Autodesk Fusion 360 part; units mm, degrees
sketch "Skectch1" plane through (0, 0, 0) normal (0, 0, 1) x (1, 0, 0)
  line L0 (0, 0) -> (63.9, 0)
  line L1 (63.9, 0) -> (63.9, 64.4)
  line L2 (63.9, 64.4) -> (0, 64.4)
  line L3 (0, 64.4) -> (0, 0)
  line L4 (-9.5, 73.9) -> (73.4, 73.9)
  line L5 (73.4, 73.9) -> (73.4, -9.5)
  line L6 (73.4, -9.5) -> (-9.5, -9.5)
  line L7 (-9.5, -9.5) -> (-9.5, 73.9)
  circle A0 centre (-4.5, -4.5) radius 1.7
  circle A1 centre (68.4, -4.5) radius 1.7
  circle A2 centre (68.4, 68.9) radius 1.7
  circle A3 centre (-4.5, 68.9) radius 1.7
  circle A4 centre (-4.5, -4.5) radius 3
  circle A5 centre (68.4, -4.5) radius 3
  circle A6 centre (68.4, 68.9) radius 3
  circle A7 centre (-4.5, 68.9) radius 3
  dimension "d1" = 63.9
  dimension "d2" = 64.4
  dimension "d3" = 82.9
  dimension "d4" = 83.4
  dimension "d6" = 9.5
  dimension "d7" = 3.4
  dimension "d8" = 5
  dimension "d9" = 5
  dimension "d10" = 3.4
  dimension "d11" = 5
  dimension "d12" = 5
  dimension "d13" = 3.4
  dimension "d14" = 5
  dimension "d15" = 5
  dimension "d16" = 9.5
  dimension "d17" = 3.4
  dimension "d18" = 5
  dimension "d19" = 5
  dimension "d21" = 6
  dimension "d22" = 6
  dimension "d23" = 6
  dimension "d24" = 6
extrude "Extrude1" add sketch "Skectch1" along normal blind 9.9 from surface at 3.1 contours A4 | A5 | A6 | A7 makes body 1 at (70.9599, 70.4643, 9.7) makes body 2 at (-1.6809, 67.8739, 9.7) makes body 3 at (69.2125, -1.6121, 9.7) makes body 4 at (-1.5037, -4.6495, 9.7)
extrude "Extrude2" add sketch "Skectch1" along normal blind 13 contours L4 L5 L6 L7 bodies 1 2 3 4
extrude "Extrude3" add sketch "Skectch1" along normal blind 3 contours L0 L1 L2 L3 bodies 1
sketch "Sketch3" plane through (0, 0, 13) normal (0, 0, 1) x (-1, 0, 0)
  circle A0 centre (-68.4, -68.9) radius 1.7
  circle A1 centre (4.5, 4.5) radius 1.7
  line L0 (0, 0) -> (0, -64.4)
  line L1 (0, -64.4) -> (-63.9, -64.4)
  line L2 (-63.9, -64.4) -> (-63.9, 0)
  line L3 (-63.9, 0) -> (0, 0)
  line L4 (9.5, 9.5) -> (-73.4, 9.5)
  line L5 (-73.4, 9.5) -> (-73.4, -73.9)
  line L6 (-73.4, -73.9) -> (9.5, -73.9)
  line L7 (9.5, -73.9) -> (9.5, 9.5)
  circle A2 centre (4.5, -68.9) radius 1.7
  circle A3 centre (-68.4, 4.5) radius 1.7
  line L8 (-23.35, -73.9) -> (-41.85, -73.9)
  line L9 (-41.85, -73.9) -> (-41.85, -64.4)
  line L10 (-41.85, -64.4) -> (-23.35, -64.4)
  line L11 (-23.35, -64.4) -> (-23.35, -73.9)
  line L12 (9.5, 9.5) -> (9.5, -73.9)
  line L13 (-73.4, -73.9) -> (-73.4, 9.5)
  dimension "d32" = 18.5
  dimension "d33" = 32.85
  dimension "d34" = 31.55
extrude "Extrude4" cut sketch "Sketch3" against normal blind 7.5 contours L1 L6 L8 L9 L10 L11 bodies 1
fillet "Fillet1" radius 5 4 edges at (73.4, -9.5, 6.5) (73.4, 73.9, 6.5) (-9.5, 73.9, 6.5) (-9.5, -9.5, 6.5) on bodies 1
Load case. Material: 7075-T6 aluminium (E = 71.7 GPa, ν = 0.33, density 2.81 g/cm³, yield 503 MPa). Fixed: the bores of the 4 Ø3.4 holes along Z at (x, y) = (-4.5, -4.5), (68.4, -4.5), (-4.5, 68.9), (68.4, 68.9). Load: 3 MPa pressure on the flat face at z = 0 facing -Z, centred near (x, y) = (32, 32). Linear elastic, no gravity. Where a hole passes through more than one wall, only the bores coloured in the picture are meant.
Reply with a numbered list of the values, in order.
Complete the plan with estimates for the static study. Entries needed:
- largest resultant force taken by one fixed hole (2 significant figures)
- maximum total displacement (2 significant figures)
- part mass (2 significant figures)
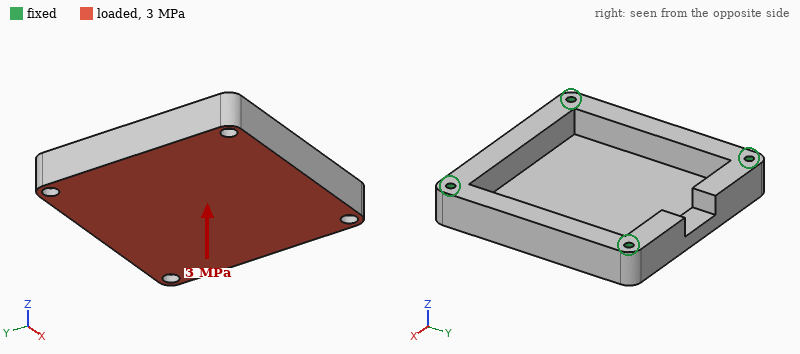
1. 7.8 kN
2. 0.64 mm
3. 130 g
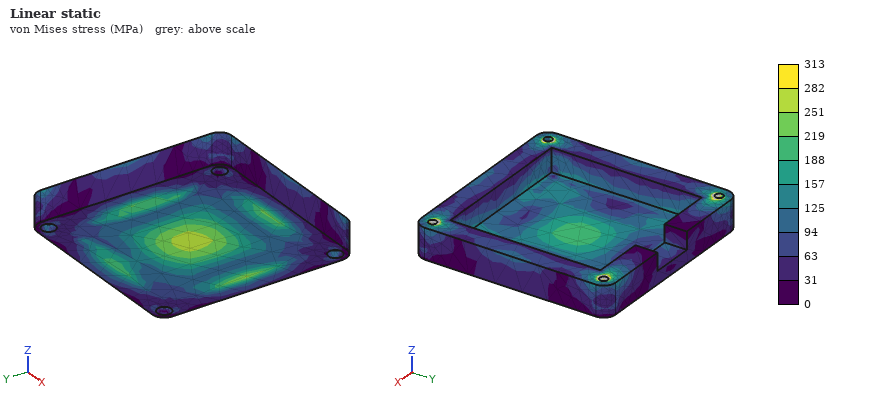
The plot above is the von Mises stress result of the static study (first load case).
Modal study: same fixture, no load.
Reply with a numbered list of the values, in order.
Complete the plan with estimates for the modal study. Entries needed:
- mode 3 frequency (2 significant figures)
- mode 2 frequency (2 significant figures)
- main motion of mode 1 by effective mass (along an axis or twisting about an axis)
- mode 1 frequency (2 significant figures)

1. 8200 Hz
2. 8100 Hz
3. along Z
4. 4800 Hz
